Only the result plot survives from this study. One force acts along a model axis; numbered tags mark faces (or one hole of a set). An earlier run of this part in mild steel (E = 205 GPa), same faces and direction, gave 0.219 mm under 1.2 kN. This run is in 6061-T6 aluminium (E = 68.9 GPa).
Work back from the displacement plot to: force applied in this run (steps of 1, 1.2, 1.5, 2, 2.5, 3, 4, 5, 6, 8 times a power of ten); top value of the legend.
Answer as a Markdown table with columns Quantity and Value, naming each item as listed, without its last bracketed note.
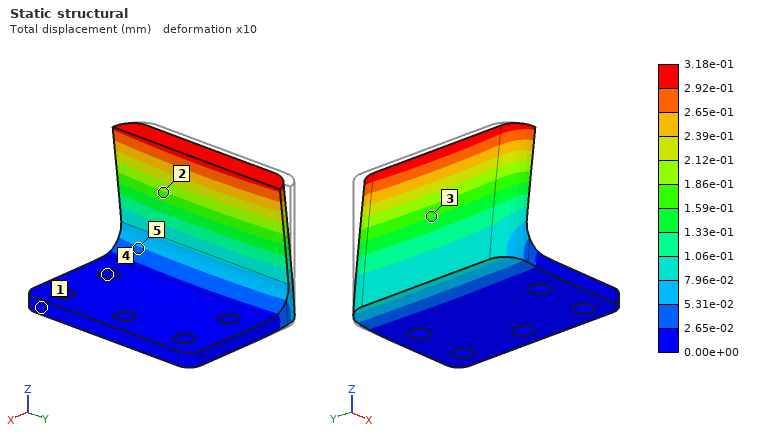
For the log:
| Quantity | Value |
|---|---|
| force applied in this run | 600 N |
| top value of the legend | 3.18e-01 mm |
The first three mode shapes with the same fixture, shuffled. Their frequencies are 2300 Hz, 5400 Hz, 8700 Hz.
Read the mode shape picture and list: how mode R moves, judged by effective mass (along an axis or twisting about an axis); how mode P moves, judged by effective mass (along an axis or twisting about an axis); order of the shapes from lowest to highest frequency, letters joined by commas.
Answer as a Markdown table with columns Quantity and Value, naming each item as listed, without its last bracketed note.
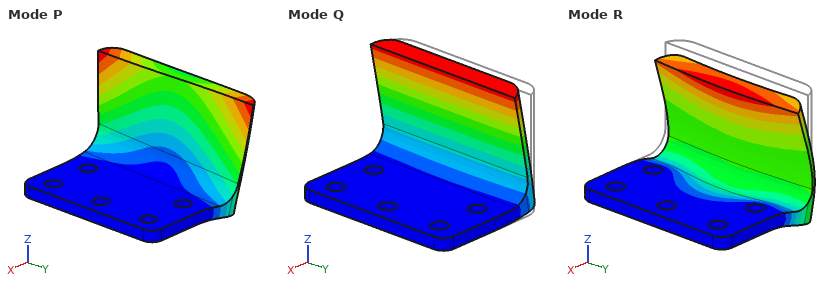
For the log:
| Quantity | Value |
|---|---|
| how mode R moves, judged by effective mass | along Z |
| how mode P moves, judged by effective mass | along Y |
| order of the shapes from lowest to highest frequency, letters joined by commas | Q, P, R |
